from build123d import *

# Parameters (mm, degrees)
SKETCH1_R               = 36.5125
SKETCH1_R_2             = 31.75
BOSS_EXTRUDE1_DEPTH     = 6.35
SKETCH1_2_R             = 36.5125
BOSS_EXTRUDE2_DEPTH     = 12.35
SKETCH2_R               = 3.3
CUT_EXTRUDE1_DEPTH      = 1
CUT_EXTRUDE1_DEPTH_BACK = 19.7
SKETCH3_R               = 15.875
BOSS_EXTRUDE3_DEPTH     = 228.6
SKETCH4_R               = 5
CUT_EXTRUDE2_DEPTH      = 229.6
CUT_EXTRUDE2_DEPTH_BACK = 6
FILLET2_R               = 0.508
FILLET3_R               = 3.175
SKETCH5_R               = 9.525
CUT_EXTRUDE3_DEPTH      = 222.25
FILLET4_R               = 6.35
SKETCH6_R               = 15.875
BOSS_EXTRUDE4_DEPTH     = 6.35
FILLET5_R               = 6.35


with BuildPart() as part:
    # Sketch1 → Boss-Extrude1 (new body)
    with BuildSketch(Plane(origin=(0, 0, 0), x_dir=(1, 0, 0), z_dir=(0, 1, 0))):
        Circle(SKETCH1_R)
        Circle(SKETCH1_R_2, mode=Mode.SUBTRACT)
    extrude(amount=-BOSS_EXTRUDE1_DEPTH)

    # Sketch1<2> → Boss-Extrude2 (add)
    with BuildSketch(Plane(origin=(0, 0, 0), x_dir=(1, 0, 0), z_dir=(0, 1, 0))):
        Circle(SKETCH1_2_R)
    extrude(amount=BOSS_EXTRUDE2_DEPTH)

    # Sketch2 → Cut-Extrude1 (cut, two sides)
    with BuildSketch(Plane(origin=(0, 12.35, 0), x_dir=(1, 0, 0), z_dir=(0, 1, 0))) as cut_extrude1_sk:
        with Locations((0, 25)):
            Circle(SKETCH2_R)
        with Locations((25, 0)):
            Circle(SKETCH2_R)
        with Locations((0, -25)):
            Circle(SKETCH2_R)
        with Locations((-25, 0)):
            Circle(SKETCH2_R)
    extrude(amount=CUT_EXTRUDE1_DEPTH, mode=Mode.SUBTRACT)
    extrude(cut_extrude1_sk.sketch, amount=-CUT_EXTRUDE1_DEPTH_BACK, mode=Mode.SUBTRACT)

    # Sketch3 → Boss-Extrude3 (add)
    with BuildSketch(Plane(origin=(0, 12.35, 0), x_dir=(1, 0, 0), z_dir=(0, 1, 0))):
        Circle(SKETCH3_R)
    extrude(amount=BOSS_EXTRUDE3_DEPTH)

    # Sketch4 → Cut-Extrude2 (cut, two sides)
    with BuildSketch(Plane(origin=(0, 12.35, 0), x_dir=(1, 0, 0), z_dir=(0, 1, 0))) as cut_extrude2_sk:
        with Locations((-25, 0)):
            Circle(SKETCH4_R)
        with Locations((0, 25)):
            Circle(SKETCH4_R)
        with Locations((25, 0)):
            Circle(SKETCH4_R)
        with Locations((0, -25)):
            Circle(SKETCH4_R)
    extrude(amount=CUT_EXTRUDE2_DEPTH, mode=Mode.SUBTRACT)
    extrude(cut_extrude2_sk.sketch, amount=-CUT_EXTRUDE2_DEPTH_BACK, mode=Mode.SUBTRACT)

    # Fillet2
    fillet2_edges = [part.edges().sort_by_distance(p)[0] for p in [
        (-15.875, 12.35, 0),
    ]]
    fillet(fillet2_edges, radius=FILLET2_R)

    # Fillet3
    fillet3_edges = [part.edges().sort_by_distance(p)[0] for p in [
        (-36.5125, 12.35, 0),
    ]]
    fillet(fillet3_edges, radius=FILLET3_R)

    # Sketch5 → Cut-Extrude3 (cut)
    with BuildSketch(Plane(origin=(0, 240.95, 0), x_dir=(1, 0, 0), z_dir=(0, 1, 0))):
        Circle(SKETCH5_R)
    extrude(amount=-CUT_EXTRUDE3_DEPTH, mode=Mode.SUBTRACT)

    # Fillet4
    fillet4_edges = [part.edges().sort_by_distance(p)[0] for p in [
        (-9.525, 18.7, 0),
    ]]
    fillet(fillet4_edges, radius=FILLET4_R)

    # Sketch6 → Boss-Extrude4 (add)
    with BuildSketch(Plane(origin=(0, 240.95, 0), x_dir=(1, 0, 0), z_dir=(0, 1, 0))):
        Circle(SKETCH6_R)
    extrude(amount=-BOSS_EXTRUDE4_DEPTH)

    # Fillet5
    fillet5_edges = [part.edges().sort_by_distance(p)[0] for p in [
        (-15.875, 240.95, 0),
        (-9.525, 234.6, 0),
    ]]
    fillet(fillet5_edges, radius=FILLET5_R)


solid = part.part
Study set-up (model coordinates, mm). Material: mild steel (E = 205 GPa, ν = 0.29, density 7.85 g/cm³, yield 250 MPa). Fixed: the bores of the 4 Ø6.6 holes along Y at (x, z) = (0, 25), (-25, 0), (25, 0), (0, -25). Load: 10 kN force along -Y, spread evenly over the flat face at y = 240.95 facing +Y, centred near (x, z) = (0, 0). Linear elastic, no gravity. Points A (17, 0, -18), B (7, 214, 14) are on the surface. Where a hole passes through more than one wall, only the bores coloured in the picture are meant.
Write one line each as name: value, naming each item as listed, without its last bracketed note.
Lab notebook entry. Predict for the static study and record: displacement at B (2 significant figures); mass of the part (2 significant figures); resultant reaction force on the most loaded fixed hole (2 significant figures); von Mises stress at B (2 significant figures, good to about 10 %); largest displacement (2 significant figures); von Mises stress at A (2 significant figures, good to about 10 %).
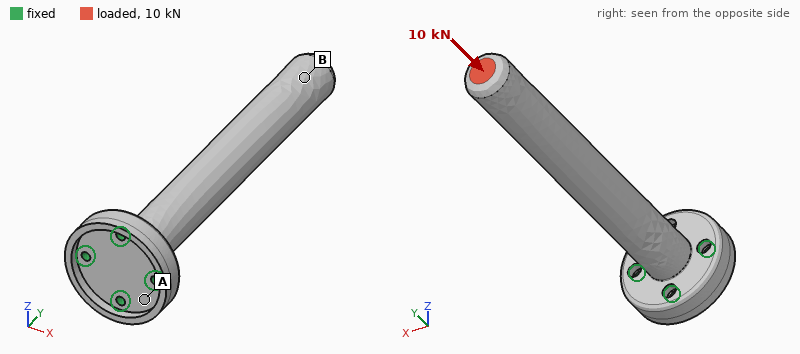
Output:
displacement at B: 22 µm
mass of the part: 1.4 kg
resultant reaction force on the most loaded fixed hole: 2.8 kN
von Mises stress at B: 21 MPa
largest displacement: 28 µm
von Mises stress at A: 8.5 MPa
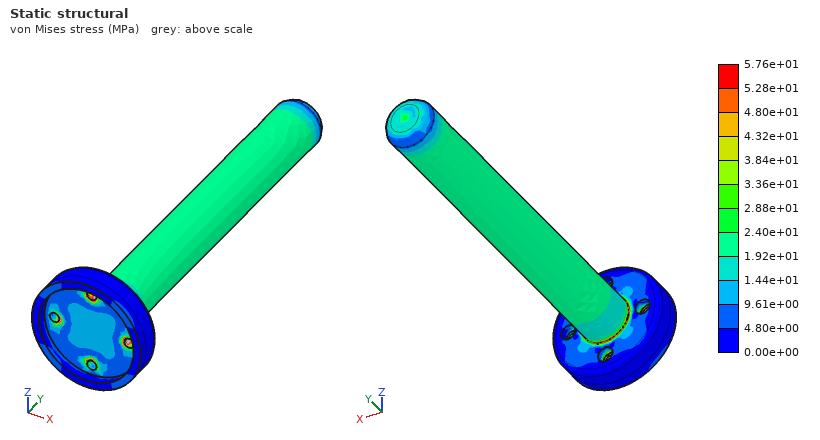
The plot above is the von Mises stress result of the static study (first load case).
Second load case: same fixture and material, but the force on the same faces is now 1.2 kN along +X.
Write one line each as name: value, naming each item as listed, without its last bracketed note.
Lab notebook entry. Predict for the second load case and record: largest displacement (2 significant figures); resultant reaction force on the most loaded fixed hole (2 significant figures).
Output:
largest displacement: 0.63 mm
resultant reaction force on the most loaded fixed hole: 5.9 kN
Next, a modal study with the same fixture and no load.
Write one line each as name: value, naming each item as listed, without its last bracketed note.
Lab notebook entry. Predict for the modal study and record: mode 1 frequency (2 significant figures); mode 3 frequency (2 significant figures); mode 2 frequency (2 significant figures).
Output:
mode 1 frequency: 440 Hz
mode 3 frequency: 2600 Hz
mode 2 frequency: 440 Hz
